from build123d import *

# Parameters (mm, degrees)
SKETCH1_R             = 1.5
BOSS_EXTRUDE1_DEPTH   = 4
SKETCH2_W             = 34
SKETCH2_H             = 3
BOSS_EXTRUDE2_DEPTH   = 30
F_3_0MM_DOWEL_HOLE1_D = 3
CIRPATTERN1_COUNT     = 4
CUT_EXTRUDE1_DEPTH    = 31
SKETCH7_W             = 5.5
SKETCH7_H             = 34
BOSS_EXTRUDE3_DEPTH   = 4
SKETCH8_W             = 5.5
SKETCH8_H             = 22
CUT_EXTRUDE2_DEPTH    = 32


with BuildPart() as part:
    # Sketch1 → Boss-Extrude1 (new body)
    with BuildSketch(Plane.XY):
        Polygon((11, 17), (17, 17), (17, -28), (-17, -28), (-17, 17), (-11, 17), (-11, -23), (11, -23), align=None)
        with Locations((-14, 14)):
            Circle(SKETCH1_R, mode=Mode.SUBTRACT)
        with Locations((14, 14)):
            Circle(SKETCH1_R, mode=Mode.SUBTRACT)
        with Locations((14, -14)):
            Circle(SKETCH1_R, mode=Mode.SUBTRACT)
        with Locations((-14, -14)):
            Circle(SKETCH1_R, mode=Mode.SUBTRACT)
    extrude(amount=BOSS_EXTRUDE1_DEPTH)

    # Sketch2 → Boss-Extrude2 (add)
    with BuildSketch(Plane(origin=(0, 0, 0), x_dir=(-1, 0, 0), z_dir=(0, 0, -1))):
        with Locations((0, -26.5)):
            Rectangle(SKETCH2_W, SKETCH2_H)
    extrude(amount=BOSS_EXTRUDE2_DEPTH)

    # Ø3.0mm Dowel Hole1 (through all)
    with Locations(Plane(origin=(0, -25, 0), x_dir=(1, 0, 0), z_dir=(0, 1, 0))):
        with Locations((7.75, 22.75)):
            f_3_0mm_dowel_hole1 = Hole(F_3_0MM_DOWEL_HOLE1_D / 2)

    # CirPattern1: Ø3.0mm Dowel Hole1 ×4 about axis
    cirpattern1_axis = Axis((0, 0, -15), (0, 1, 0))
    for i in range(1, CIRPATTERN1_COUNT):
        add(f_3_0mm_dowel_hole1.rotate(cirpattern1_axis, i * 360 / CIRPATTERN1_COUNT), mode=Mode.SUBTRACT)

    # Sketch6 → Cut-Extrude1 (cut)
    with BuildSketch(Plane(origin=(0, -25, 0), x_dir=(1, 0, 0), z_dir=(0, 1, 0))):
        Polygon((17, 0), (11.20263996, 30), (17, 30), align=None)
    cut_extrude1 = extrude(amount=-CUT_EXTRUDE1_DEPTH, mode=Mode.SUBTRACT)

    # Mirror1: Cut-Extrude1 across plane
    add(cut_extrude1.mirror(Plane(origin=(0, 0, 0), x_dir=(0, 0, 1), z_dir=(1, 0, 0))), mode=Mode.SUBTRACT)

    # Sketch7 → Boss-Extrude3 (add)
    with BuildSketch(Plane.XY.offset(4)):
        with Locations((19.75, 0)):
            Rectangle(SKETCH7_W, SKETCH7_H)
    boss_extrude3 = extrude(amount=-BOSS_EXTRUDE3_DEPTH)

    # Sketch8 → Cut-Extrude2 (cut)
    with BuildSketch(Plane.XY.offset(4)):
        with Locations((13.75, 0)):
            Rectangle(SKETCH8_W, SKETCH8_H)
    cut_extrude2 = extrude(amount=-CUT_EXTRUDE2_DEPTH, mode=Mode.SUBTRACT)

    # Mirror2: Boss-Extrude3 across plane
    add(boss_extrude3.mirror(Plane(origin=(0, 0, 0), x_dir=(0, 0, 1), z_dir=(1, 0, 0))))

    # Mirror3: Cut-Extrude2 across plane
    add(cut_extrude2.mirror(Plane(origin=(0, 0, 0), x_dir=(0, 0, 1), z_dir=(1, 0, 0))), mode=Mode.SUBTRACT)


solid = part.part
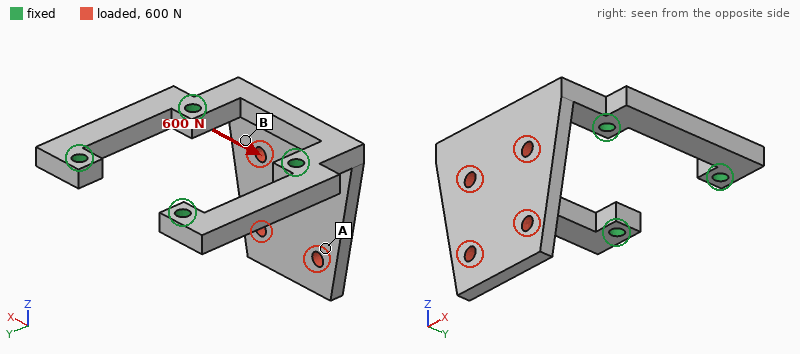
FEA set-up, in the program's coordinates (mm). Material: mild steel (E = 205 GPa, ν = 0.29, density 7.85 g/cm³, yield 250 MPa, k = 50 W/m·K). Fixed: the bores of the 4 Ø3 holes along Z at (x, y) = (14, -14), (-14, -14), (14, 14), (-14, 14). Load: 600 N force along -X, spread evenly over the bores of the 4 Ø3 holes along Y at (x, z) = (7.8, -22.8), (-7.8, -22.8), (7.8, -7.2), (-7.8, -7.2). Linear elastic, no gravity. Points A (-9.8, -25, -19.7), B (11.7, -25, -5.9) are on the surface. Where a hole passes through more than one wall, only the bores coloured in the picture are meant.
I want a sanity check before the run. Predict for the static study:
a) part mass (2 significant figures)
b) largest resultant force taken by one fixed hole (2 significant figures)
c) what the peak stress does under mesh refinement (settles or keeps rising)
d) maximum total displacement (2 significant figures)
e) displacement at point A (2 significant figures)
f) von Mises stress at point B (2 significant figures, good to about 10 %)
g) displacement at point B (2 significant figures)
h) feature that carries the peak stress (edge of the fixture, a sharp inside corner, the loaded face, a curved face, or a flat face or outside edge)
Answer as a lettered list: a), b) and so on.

a) 43 g
b) 460 N
c) keeps rising
d) 46 µm
e) 34 µm
f) 45 MPa
g) 20 µm
h) edge of the fixture
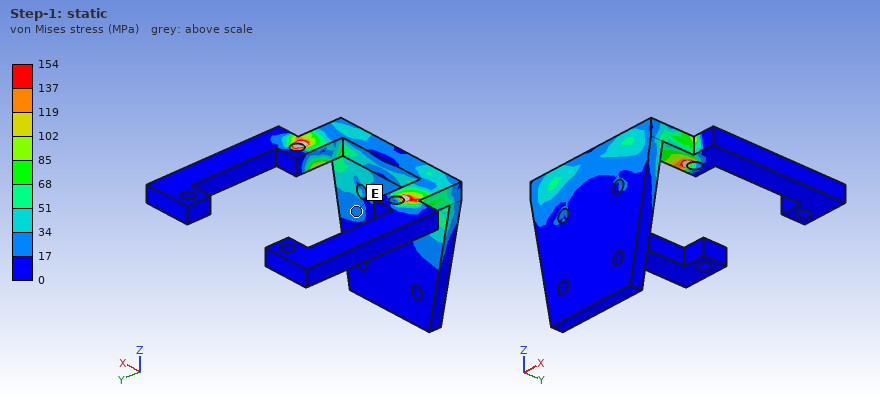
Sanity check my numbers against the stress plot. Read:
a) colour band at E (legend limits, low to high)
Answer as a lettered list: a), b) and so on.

a) 17 to 34 MPa
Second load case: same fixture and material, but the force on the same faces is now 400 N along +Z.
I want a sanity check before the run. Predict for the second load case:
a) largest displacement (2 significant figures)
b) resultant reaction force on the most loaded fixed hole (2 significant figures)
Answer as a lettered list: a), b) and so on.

a) 68 µm
b) 200 N
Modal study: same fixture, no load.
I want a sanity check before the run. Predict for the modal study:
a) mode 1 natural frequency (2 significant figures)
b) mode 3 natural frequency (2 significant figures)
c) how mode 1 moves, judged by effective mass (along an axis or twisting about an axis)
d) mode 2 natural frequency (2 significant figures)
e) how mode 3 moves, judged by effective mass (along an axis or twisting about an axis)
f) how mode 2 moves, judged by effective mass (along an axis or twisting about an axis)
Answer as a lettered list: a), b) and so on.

a) 1700 Hz
b) 6500 Hz
c) along Y
d) 4800 Hz
e) along Z
f) along X
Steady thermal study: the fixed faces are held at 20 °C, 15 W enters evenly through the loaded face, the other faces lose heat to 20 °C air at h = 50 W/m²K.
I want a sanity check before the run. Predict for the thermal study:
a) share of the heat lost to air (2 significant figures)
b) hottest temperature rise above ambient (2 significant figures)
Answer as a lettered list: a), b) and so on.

a) 47 %
b) 78 K
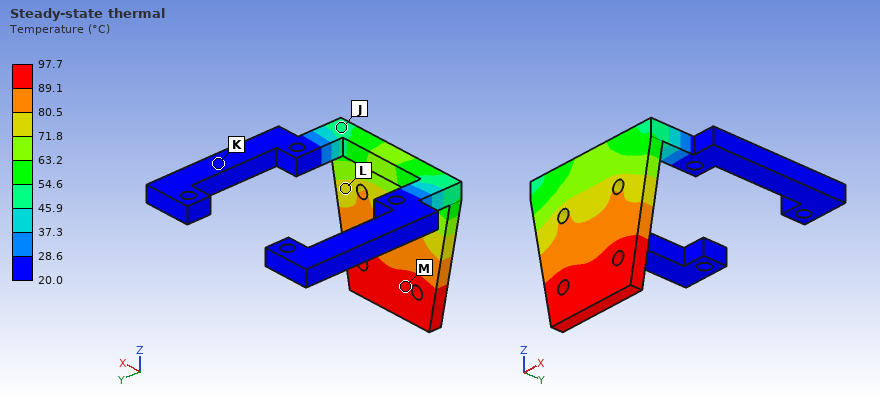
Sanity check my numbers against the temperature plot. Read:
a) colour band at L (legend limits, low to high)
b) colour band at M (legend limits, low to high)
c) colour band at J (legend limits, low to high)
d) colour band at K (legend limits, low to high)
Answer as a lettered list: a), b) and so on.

a) 71.8 to 80.5 °C
b) 89.1 to 97.7 °C
c) 45.9 to 54.6 °C
d) 20.0 to 28.6 °C
